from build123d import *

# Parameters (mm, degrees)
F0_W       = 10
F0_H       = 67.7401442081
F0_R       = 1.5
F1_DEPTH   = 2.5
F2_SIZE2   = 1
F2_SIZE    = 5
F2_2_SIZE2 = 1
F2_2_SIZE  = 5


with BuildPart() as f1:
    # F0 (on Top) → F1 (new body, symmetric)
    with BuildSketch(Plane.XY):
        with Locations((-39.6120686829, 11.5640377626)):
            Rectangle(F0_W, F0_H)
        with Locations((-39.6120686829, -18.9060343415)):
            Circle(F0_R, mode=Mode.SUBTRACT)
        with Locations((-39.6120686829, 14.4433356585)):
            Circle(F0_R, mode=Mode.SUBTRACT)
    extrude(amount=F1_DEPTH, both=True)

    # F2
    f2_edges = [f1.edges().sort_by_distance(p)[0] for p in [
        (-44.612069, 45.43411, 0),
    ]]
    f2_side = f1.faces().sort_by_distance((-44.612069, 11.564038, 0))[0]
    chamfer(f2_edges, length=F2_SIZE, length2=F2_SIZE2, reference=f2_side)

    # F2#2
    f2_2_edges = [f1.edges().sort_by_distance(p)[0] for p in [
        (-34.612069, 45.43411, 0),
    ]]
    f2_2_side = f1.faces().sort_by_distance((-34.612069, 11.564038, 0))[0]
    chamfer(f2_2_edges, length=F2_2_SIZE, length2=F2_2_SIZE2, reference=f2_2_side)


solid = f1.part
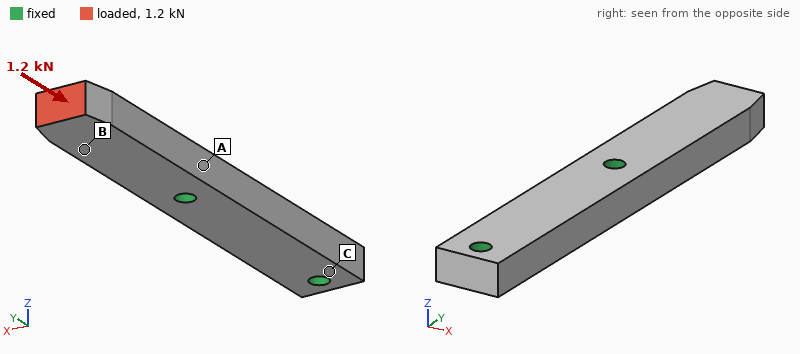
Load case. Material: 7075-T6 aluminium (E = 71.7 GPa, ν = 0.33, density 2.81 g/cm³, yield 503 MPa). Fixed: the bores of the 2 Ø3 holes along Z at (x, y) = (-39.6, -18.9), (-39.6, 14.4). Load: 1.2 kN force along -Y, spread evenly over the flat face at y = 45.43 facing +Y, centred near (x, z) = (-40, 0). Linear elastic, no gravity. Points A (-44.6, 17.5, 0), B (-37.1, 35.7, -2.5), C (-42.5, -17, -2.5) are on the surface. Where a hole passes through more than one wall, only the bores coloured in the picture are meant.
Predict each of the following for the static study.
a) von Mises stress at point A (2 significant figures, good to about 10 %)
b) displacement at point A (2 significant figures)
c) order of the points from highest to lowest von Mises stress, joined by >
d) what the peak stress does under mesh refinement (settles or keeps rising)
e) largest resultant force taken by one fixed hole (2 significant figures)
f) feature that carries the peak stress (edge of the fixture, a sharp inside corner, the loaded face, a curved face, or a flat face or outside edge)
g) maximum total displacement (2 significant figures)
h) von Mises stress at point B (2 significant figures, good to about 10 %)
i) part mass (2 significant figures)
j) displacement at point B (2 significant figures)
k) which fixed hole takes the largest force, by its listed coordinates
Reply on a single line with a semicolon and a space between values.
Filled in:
14 MPa; 1.7 µm; B > A > C; keeps rising; 1.2 kN; edge of the fixture; 11 µm; 24 MPa; 9.2 g; 7.4 µm; (-39.6, 14.4)
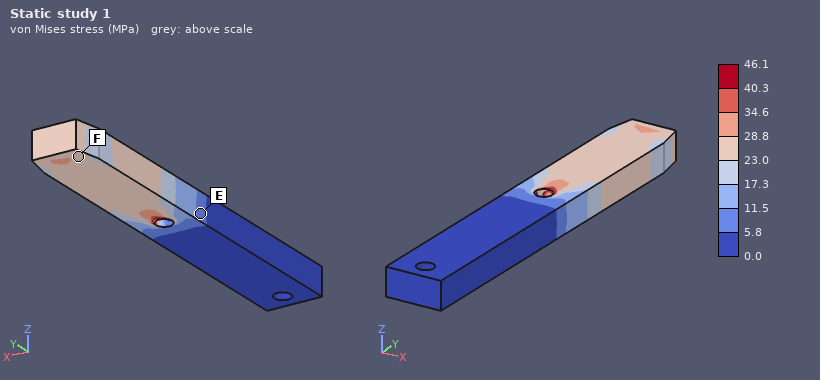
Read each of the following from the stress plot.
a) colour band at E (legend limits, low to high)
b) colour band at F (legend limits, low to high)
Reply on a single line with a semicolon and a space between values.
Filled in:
5.8 to 11.5 MPa; 23.0 to 28.8 MPa
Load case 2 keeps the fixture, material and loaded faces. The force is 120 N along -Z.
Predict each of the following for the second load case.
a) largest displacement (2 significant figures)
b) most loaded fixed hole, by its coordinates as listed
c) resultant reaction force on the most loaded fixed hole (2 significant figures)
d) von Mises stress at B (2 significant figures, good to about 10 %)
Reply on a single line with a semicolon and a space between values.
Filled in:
0.16 mm; (-39.6, 14.4); 130 N; 28 MPa
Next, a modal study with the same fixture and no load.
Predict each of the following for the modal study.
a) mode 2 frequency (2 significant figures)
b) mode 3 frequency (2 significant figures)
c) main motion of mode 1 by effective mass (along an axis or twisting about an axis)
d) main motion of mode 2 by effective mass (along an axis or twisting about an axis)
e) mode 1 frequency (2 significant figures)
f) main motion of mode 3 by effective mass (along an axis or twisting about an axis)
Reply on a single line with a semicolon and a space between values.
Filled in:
6700 Hz; 20 kHz; along Z; along X; 4400 Hz; twisting about Y
